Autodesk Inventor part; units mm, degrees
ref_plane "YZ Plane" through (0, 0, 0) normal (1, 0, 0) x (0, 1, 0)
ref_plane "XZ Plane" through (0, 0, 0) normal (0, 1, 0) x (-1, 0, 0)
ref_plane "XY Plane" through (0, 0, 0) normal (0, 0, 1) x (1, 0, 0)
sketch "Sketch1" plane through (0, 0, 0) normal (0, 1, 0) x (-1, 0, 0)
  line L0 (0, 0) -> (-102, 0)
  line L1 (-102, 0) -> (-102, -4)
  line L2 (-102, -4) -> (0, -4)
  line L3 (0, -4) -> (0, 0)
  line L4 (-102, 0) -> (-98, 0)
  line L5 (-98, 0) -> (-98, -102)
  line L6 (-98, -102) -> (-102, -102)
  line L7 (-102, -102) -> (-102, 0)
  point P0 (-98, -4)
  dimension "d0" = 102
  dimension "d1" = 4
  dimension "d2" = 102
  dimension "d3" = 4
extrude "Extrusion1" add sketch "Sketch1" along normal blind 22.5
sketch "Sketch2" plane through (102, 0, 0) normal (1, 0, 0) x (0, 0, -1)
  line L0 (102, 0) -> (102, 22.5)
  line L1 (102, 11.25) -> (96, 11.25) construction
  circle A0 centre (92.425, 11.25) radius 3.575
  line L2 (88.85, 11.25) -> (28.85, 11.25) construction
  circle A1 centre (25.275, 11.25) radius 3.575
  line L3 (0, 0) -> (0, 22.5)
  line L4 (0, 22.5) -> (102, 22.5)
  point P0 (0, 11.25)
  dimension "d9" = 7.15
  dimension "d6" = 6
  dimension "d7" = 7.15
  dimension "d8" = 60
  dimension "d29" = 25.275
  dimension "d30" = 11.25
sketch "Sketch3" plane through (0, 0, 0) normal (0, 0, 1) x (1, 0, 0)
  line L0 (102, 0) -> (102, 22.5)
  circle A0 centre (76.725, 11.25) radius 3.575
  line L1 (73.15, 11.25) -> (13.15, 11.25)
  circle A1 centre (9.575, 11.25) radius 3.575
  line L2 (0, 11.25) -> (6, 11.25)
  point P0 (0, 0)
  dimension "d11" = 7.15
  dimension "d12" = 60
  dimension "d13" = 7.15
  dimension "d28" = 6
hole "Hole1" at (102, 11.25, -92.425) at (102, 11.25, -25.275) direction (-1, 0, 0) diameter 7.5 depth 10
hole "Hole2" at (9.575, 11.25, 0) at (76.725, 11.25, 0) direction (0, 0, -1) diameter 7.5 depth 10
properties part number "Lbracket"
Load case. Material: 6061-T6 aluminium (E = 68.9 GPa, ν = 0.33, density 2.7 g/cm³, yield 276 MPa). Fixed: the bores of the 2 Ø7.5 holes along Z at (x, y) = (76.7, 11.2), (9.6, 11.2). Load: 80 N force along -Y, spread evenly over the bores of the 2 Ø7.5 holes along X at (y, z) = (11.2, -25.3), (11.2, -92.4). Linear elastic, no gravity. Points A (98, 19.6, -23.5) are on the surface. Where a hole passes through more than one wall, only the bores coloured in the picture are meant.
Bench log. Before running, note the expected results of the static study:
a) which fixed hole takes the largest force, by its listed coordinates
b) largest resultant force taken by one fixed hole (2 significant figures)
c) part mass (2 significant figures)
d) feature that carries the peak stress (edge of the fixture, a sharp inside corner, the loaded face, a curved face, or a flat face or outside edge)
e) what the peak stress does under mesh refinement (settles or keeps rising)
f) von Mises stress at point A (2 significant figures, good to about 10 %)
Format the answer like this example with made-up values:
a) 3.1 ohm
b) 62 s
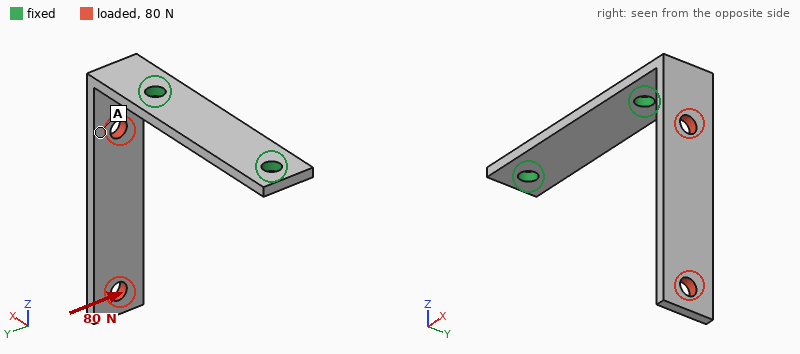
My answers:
a) (76.7, 11.2)
b) 91 N
c) 47 g
d) edge of the fixture
e) keeps rising
f) 8.1 MPa
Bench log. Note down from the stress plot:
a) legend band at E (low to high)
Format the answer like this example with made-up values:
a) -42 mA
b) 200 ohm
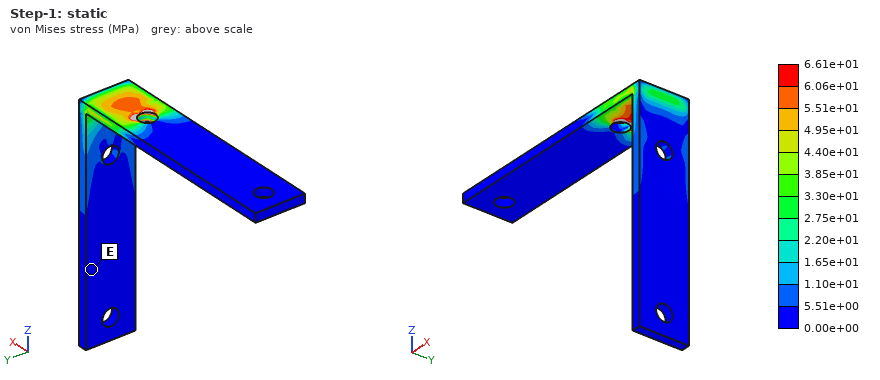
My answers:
a) 0.00e+00 to 5.51e+00 MPa
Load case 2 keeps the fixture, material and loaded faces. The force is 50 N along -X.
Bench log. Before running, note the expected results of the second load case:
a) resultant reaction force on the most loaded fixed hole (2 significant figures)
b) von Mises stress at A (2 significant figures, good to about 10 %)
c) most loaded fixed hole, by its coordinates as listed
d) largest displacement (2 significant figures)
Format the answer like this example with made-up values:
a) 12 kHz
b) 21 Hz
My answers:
a) 48 N
b) 40 MPa
c) (76.7, 11.2)
d) 1.6 mm
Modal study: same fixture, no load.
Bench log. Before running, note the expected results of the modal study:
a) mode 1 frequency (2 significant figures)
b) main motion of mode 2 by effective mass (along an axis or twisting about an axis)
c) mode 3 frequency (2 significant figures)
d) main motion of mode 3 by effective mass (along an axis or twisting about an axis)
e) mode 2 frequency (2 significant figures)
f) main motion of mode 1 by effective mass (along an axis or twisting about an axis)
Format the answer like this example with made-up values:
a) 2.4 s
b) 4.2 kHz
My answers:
a) 250 Hz
b) along Y
c) 1500 Hz
d) along Z
e) 460 Hz
f) along X
